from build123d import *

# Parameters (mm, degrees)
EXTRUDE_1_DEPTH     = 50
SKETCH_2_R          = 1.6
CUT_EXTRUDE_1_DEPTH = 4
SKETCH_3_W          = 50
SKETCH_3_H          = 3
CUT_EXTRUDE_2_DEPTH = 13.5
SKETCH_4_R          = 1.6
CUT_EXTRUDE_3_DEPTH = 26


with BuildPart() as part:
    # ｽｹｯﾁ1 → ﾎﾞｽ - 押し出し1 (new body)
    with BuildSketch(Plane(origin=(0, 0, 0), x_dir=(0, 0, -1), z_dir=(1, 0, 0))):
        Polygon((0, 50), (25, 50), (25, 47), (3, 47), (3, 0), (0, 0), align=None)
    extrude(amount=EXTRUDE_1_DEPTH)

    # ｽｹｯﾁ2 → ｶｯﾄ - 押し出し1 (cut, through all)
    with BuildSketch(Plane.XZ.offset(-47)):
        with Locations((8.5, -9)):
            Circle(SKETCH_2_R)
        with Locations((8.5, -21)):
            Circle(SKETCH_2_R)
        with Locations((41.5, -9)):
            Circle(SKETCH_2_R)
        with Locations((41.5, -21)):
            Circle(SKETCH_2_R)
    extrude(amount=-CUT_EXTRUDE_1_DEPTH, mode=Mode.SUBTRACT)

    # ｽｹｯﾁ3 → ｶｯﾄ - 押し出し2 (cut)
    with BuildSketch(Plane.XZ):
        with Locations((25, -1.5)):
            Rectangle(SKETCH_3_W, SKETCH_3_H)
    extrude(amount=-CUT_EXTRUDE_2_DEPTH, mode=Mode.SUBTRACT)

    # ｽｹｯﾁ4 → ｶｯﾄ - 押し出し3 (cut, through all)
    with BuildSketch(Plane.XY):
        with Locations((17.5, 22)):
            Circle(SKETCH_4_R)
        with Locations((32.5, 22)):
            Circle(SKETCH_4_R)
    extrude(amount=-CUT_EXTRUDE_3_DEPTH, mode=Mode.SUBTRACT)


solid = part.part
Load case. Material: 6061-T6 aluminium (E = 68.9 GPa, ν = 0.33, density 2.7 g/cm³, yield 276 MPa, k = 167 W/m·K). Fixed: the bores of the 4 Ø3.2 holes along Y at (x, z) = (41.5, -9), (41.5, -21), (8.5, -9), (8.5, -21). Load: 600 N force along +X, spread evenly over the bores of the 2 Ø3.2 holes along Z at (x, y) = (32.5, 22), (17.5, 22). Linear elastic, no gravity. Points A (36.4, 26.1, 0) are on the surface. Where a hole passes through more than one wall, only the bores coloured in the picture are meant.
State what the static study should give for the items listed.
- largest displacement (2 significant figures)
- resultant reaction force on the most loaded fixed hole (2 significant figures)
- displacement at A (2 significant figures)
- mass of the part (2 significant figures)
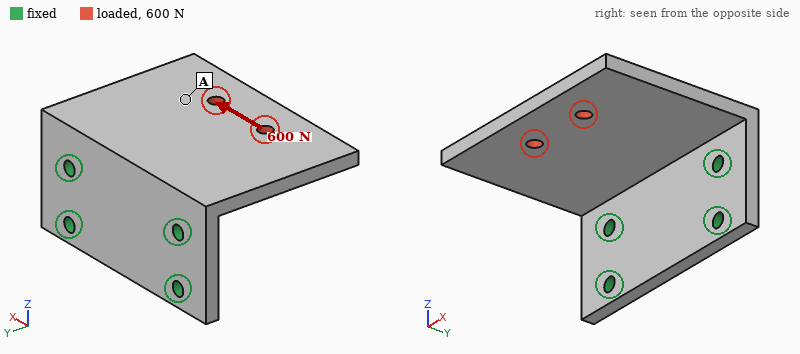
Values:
76 µm
580 N
37 µm
23 g
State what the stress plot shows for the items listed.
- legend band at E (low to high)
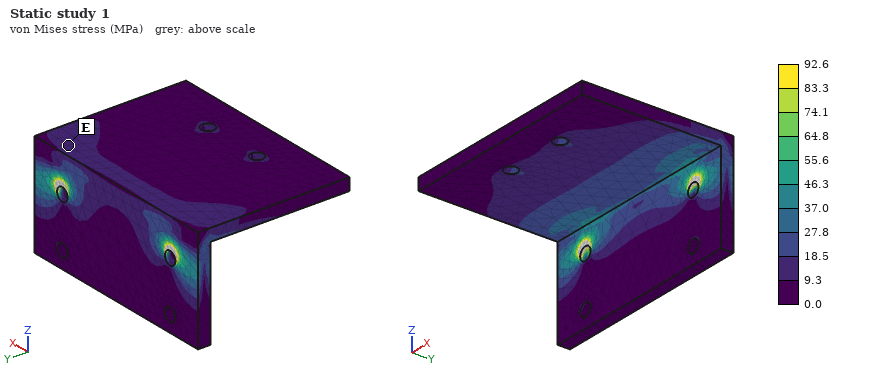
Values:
9.3 to 18.5 MPa
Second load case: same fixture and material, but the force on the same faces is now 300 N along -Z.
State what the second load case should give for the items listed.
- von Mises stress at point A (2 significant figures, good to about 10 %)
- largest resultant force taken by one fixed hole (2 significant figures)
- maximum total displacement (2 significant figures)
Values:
24 MPa
180 N
0.60 mm
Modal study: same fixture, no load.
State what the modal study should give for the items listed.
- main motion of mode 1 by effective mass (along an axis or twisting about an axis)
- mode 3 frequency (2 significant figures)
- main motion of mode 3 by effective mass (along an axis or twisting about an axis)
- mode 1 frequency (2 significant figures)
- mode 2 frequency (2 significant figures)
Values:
along Z
6500 Hz
along X
1500 Hz
3200 Hz
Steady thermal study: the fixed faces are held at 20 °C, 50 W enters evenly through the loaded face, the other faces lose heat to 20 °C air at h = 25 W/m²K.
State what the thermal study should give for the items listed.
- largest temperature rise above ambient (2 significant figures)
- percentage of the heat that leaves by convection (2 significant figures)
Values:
80 K
10.0 %
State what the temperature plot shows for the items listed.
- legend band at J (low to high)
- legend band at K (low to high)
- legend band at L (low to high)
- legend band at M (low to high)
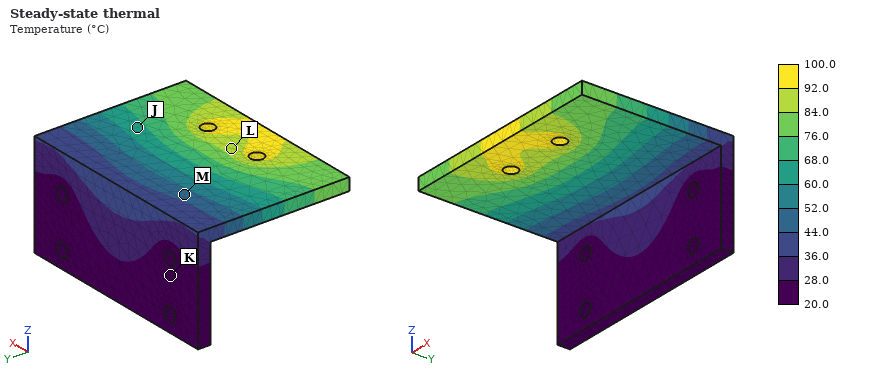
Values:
60.0 to 68.0 °C
20.0 to 28.0 °C
84.0 to 92.0 °C
44.0 to 52.0 °C
